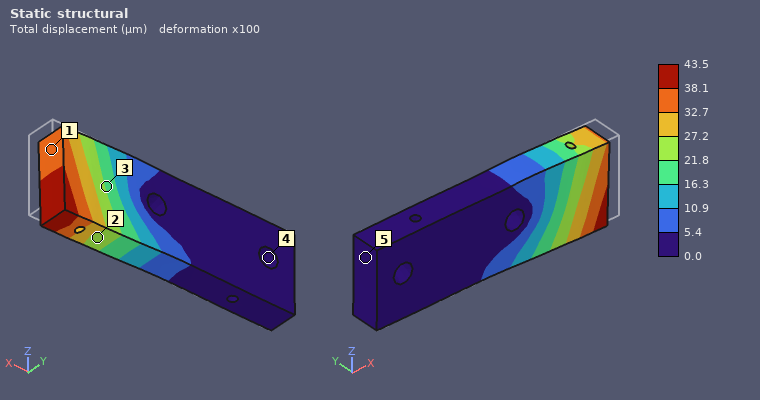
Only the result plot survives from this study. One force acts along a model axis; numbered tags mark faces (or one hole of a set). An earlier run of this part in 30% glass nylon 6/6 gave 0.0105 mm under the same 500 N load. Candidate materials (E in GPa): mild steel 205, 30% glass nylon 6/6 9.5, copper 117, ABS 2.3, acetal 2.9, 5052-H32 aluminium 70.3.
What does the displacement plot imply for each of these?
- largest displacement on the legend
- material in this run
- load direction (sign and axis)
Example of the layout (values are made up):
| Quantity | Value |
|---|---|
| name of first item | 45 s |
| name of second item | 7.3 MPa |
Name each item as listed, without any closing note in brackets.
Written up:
| Quantity | Value |
|---|---|
| largest displacement on the legend | 43.5 µm |
| material in this run | ABS |
| load direction | -X |
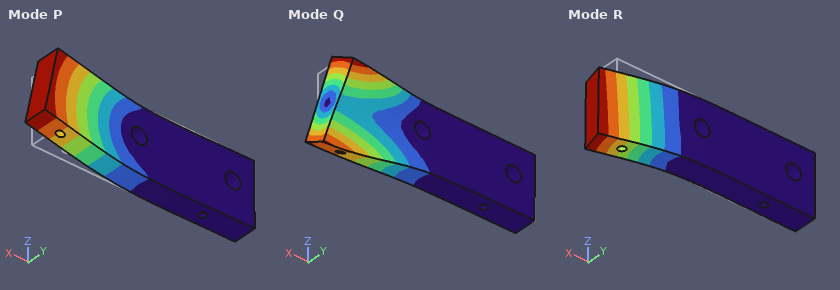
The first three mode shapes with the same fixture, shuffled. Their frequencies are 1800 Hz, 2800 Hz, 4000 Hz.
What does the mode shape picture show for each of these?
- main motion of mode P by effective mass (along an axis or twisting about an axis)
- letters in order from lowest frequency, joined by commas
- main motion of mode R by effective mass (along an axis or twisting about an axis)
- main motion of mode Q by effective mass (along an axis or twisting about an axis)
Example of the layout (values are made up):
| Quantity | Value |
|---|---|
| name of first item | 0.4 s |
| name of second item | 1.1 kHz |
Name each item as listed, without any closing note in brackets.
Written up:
| Quantity | Value |
|---|---|
| main motion of mode P by effective mass | along Z |
| letters in order from lowest frequency, joined by commas | R, P, Q |
| main motion of mode R by effective mass | along Y |
| main motion of mode Q by effective mass | twisting about X |
